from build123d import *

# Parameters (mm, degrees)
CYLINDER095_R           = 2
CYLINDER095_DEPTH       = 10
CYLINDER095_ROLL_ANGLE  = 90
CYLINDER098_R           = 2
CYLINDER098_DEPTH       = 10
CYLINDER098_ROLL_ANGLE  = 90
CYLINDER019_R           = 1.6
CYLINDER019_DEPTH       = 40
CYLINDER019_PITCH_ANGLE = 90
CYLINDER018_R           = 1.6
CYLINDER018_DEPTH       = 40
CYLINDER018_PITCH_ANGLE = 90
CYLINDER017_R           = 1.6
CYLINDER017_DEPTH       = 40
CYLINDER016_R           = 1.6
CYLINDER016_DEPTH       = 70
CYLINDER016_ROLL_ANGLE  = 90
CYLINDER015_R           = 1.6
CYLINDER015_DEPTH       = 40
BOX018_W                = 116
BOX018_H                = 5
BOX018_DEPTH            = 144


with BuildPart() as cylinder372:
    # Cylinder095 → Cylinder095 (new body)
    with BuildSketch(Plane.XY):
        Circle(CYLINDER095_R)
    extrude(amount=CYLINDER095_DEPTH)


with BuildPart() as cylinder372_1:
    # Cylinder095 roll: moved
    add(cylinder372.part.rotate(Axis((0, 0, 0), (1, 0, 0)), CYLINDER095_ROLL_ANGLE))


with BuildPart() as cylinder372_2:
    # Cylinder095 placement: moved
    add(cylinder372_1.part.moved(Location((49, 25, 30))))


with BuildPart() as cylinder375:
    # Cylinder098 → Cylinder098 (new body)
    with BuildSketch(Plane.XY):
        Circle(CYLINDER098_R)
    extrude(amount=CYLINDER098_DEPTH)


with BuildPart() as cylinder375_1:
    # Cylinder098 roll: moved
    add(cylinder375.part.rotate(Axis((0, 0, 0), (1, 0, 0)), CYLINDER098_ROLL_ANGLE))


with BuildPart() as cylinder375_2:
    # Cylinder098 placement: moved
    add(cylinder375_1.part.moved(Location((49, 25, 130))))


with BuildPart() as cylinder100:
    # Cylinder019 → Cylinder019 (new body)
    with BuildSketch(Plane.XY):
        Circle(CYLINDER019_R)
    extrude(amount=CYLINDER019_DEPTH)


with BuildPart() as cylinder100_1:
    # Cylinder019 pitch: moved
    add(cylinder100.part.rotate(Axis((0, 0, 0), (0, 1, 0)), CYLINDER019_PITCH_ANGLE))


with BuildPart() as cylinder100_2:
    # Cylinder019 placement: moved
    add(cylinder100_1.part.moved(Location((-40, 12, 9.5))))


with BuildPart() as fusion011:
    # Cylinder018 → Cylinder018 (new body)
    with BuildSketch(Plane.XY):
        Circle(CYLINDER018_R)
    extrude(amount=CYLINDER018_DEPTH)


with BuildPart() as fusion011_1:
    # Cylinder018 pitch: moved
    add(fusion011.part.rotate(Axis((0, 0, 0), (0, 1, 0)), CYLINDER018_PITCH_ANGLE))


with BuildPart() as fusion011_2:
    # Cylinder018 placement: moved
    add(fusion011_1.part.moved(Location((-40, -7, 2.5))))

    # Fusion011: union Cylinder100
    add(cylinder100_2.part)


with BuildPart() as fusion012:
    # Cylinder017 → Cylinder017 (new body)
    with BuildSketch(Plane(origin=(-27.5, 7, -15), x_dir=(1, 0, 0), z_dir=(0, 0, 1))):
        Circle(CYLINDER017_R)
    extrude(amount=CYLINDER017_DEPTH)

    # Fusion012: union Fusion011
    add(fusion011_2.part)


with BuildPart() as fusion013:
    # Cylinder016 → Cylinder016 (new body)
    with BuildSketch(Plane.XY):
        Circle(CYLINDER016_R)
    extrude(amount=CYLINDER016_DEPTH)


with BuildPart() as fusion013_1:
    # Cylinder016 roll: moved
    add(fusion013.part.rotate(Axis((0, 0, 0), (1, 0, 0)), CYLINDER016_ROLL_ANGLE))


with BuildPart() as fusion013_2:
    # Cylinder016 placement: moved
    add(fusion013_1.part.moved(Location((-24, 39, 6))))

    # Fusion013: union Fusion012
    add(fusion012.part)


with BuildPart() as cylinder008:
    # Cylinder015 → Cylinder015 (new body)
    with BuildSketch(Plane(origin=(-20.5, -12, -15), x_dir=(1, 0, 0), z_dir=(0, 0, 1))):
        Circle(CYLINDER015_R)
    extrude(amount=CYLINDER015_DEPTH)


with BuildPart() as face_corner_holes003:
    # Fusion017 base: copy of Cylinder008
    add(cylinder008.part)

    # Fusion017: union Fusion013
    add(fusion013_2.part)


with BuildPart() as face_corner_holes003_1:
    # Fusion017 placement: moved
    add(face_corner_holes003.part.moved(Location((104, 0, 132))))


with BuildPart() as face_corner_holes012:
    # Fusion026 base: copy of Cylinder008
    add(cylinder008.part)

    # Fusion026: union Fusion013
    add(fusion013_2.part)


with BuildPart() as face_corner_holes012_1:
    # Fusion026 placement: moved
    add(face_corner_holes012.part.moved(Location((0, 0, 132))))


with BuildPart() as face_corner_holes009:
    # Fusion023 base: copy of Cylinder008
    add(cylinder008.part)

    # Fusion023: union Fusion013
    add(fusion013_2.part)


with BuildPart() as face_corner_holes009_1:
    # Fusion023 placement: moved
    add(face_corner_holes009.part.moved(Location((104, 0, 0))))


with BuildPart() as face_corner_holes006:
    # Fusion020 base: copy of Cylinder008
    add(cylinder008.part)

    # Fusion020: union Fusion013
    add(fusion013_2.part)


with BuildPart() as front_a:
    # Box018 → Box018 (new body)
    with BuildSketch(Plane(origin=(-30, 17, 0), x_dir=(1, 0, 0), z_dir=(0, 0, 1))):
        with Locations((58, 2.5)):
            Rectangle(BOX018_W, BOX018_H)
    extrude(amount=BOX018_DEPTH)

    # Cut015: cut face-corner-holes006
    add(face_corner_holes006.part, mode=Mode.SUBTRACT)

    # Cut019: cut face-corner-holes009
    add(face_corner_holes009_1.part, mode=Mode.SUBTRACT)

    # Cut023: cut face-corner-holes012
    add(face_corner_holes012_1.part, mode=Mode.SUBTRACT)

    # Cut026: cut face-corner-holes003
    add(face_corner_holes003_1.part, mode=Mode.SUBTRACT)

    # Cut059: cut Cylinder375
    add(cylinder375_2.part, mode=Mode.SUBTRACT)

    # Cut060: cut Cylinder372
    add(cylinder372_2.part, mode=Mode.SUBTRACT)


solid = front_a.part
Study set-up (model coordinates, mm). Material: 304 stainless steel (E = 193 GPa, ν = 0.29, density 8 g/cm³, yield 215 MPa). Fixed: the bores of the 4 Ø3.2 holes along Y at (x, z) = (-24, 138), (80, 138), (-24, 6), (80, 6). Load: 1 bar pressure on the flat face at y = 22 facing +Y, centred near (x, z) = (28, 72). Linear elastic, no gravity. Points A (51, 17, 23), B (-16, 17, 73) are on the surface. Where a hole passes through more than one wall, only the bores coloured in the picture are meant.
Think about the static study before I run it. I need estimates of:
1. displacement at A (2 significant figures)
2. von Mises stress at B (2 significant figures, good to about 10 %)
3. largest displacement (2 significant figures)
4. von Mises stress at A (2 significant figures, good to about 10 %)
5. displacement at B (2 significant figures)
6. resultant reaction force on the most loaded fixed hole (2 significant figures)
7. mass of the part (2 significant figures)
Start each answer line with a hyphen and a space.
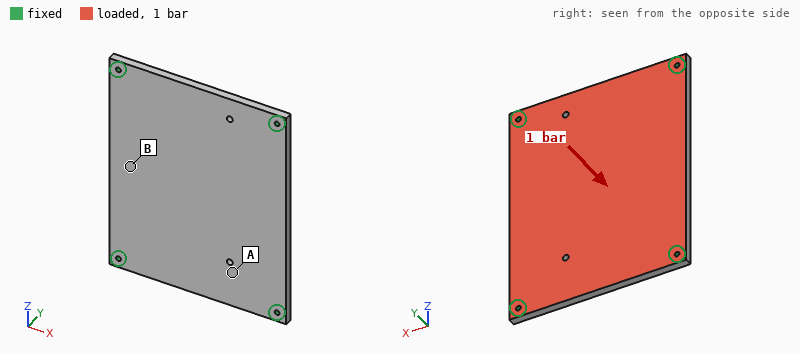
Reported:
- 45 µm
- 26 MPa
- 93 µm
- 12 MPa
- 77 µm
- 420 N
- 670 g
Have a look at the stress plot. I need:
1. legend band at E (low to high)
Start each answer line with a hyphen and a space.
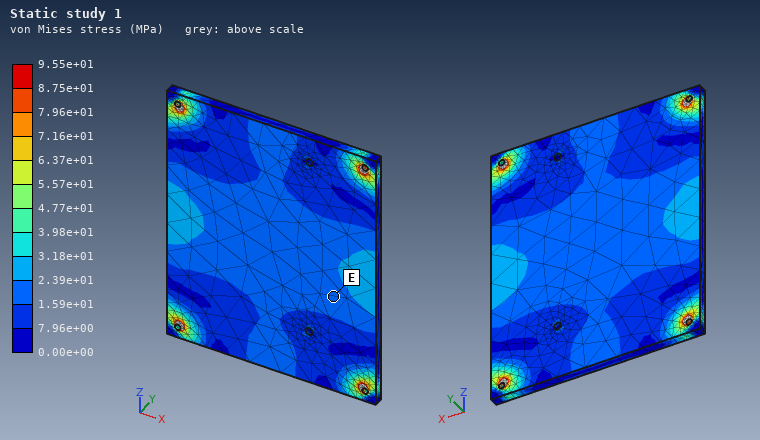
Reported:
- 1.59e+01 to 2.39e+01 MPa
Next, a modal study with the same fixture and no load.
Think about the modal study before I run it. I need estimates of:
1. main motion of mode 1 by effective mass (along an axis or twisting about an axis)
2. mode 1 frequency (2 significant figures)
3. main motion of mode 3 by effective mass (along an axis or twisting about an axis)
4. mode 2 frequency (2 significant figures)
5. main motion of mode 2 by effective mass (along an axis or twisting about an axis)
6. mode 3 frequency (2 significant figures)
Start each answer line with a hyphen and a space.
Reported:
- along Y
- 970 Hz
- twisting about X
- 1700 Hz
- twisting about Z
- 2100 Hz
